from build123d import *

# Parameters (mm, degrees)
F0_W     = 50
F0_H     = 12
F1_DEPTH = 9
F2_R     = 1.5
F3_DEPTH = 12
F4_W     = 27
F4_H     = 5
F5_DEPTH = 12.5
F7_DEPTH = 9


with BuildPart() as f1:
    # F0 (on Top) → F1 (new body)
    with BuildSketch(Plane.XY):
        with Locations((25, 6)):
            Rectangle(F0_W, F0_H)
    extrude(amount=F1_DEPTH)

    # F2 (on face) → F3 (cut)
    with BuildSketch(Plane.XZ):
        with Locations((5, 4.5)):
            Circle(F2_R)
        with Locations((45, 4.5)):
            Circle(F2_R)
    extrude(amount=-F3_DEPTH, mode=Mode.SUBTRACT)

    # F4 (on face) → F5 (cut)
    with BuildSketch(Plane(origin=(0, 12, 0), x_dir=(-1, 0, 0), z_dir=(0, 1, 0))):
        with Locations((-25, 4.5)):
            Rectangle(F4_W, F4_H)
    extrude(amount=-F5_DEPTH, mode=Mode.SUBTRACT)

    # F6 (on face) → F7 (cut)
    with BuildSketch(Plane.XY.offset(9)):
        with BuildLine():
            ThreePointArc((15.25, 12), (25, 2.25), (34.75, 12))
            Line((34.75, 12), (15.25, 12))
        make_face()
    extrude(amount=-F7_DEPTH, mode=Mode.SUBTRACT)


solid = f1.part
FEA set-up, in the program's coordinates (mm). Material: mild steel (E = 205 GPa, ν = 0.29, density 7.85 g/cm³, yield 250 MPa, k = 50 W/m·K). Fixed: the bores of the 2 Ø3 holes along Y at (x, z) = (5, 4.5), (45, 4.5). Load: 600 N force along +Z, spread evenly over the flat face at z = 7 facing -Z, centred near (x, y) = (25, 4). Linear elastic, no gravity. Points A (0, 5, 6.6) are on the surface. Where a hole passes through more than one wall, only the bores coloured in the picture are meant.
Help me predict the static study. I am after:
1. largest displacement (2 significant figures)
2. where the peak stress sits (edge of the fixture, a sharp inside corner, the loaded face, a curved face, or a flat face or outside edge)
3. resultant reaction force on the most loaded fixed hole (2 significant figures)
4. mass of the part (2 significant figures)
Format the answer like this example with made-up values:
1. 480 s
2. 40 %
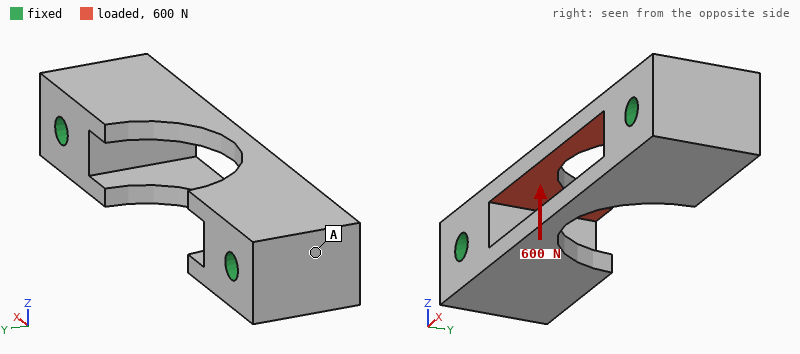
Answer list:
1. 38 µm
2. a curved face
3. 300 N
4. 24 g
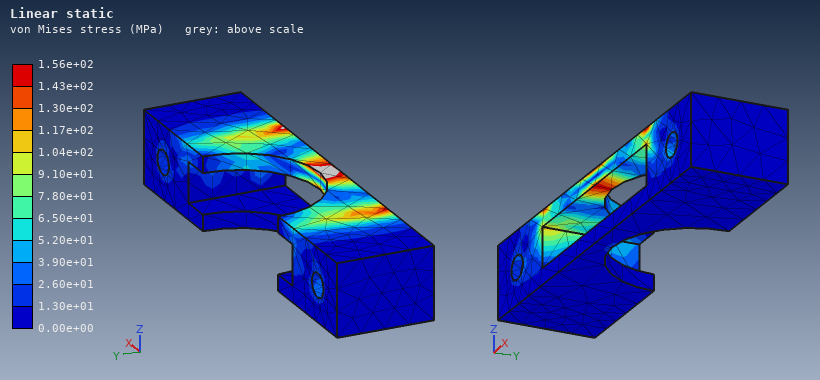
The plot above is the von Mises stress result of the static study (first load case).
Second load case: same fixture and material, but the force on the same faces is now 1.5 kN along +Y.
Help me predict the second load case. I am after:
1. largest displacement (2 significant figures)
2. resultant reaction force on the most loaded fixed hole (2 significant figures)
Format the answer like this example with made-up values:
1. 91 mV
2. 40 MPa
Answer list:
1. 17 µm
2. 790 N
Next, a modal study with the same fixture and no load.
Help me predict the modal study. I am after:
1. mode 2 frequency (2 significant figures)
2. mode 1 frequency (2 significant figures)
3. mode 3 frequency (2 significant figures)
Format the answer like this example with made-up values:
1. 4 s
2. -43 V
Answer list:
1. 16 kHz
2. 15 kHz
3. 29 kHz
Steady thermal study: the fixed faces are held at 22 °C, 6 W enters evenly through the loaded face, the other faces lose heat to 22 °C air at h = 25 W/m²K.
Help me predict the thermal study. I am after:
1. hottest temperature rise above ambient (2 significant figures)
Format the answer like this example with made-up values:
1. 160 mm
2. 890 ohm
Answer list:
1. 27 K
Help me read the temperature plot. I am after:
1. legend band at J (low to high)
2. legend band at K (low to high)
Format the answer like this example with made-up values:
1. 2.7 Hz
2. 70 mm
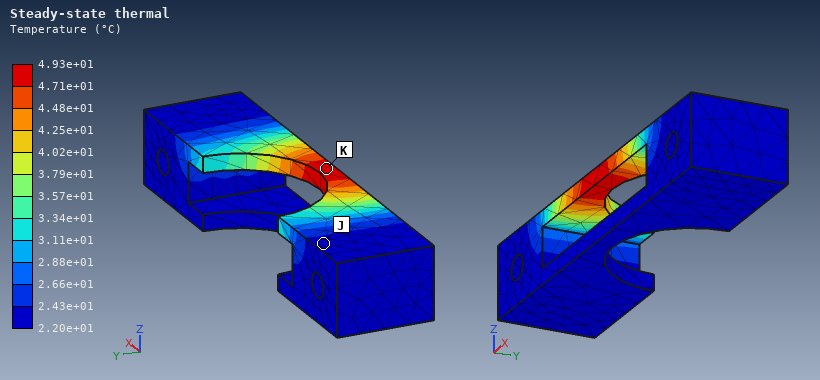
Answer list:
1. 2.20e+01 to 2.43e+01 °C
2. 4.71e+01 to 4.93e+01 °C
